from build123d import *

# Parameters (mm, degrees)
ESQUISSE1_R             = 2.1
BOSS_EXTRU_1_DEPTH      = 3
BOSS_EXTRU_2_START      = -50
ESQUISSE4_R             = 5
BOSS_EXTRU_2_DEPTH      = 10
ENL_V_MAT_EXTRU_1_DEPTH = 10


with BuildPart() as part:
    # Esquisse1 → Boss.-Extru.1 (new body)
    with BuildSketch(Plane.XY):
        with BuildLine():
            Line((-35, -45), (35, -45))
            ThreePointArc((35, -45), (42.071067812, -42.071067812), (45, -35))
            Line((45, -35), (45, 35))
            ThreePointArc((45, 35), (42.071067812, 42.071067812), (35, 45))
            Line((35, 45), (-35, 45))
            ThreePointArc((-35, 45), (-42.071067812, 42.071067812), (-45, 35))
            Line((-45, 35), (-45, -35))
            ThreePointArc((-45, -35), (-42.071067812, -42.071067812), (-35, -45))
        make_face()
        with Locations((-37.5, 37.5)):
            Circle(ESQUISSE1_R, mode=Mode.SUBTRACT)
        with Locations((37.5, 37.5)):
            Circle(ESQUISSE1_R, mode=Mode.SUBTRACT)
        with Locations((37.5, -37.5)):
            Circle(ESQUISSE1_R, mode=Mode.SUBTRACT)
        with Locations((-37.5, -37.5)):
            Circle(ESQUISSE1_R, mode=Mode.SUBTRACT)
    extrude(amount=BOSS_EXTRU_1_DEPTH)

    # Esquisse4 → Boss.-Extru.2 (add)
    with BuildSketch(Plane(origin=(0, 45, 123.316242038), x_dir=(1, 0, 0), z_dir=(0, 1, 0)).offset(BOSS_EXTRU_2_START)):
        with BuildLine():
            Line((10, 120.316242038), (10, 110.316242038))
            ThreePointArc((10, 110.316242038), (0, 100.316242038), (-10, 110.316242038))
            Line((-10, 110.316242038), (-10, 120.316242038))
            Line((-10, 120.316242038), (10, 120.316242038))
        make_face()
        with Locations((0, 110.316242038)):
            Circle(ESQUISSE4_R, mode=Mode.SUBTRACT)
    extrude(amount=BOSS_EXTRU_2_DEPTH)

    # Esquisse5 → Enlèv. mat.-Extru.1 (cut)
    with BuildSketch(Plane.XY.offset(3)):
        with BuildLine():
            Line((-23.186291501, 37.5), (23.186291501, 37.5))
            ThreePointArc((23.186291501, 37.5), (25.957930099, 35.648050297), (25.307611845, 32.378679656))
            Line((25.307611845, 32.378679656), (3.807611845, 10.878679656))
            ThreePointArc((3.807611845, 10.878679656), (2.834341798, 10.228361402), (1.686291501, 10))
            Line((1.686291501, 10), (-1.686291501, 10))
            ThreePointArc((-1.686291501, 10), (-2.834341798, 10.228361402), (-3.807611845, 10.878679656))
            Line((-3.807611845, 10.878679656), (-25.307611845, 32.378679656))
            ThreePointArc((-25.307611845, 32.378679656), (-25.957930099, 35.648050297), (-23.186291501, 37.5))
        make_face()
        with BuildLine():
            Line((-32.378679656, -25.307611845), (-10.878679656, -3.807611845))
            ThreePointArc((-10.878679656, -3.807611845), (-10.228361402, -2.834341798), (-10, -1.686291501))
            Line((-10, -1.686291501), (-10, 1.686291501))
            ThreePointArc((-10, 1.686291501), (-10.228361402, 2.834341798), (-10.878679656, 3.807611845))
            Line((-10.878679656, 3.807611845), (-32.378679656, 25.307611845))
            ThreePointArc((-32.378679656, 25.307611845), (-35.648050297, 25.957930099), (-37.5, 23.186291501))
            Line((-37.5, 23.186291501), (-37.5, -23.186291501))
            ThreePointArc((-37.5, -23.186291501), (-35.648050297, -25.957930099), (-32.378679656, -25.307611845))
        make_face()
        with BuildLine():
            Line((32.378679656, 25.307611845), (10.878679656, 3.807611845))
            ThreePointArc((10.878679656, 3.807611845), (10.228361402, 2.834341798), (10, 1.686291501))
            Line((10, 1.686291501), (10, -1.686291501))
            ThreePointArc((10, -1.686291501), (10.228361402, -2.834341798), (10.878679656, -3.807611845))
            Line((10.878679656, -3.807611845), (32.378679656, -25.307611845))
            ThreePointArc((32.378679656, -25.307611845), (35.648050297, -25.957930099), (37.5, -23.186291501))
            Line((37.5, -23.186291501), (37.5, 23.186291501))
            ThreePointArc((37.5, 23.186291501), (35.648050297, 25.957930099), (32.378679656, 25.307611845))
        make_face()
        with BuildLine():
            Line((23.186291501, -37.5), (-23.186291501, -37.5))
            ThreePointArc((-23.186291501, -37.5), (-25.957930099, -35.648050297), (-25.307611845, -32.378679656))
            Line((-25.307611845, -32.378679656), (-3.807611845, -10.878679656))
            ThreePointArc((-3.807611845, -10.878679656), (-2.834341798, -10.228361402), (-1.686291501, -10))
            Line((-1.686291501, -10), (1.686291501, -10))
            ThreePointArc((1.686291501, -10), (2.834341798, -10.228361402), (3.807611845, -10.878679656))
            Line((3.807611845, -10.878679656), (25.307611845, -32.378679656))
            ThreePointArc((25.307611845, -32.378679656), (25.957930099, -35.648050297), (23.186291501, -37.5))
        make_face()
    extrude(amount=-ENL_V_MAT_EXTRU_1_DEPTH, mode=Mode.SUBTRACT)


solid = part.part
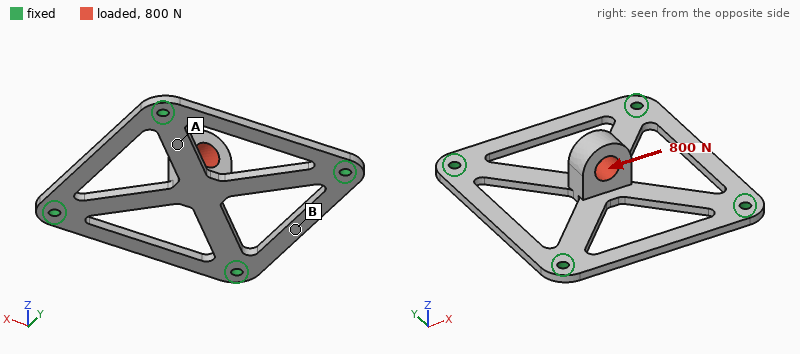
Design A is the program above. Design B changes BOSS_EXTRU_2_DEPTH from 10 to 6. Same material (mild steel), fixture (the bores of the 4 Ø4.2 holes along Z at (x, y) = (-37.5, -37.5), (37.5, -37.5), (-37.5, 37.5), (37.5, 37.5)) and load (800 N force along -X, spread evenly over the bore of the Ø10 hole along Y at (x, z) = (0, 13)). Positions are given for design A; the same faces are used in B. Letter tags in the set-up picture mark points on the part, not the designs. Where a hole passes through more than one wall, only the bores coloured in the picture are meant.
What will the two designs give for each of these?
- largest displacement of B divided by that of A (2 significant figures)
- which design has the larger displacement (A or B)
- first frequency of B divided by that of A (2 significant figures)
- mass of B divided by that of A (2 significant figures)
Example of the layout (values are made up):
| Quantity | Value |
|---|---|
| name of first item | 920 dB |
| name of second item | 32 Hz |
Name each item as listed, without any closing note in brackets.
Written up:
| Quantity | Value |
|---|---|
| largest displacement of B divided by that of A | 1.1 |
| which design has the larger displacement | B |
| first frequency of B divided by that of A | 1.1 |
| mass of B divided by that of A | 0.93 |
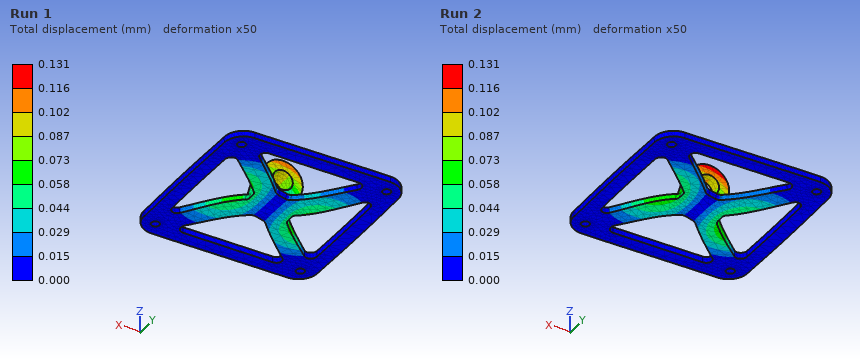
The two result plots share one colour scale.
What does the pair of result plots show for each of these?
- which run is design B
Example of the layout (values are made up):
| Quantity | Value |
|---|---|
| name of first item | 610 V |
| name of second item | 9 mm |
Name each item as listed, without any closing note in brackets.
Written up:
| Quantity | Value |
|---|---|
| which run is design B | Run 2 |
